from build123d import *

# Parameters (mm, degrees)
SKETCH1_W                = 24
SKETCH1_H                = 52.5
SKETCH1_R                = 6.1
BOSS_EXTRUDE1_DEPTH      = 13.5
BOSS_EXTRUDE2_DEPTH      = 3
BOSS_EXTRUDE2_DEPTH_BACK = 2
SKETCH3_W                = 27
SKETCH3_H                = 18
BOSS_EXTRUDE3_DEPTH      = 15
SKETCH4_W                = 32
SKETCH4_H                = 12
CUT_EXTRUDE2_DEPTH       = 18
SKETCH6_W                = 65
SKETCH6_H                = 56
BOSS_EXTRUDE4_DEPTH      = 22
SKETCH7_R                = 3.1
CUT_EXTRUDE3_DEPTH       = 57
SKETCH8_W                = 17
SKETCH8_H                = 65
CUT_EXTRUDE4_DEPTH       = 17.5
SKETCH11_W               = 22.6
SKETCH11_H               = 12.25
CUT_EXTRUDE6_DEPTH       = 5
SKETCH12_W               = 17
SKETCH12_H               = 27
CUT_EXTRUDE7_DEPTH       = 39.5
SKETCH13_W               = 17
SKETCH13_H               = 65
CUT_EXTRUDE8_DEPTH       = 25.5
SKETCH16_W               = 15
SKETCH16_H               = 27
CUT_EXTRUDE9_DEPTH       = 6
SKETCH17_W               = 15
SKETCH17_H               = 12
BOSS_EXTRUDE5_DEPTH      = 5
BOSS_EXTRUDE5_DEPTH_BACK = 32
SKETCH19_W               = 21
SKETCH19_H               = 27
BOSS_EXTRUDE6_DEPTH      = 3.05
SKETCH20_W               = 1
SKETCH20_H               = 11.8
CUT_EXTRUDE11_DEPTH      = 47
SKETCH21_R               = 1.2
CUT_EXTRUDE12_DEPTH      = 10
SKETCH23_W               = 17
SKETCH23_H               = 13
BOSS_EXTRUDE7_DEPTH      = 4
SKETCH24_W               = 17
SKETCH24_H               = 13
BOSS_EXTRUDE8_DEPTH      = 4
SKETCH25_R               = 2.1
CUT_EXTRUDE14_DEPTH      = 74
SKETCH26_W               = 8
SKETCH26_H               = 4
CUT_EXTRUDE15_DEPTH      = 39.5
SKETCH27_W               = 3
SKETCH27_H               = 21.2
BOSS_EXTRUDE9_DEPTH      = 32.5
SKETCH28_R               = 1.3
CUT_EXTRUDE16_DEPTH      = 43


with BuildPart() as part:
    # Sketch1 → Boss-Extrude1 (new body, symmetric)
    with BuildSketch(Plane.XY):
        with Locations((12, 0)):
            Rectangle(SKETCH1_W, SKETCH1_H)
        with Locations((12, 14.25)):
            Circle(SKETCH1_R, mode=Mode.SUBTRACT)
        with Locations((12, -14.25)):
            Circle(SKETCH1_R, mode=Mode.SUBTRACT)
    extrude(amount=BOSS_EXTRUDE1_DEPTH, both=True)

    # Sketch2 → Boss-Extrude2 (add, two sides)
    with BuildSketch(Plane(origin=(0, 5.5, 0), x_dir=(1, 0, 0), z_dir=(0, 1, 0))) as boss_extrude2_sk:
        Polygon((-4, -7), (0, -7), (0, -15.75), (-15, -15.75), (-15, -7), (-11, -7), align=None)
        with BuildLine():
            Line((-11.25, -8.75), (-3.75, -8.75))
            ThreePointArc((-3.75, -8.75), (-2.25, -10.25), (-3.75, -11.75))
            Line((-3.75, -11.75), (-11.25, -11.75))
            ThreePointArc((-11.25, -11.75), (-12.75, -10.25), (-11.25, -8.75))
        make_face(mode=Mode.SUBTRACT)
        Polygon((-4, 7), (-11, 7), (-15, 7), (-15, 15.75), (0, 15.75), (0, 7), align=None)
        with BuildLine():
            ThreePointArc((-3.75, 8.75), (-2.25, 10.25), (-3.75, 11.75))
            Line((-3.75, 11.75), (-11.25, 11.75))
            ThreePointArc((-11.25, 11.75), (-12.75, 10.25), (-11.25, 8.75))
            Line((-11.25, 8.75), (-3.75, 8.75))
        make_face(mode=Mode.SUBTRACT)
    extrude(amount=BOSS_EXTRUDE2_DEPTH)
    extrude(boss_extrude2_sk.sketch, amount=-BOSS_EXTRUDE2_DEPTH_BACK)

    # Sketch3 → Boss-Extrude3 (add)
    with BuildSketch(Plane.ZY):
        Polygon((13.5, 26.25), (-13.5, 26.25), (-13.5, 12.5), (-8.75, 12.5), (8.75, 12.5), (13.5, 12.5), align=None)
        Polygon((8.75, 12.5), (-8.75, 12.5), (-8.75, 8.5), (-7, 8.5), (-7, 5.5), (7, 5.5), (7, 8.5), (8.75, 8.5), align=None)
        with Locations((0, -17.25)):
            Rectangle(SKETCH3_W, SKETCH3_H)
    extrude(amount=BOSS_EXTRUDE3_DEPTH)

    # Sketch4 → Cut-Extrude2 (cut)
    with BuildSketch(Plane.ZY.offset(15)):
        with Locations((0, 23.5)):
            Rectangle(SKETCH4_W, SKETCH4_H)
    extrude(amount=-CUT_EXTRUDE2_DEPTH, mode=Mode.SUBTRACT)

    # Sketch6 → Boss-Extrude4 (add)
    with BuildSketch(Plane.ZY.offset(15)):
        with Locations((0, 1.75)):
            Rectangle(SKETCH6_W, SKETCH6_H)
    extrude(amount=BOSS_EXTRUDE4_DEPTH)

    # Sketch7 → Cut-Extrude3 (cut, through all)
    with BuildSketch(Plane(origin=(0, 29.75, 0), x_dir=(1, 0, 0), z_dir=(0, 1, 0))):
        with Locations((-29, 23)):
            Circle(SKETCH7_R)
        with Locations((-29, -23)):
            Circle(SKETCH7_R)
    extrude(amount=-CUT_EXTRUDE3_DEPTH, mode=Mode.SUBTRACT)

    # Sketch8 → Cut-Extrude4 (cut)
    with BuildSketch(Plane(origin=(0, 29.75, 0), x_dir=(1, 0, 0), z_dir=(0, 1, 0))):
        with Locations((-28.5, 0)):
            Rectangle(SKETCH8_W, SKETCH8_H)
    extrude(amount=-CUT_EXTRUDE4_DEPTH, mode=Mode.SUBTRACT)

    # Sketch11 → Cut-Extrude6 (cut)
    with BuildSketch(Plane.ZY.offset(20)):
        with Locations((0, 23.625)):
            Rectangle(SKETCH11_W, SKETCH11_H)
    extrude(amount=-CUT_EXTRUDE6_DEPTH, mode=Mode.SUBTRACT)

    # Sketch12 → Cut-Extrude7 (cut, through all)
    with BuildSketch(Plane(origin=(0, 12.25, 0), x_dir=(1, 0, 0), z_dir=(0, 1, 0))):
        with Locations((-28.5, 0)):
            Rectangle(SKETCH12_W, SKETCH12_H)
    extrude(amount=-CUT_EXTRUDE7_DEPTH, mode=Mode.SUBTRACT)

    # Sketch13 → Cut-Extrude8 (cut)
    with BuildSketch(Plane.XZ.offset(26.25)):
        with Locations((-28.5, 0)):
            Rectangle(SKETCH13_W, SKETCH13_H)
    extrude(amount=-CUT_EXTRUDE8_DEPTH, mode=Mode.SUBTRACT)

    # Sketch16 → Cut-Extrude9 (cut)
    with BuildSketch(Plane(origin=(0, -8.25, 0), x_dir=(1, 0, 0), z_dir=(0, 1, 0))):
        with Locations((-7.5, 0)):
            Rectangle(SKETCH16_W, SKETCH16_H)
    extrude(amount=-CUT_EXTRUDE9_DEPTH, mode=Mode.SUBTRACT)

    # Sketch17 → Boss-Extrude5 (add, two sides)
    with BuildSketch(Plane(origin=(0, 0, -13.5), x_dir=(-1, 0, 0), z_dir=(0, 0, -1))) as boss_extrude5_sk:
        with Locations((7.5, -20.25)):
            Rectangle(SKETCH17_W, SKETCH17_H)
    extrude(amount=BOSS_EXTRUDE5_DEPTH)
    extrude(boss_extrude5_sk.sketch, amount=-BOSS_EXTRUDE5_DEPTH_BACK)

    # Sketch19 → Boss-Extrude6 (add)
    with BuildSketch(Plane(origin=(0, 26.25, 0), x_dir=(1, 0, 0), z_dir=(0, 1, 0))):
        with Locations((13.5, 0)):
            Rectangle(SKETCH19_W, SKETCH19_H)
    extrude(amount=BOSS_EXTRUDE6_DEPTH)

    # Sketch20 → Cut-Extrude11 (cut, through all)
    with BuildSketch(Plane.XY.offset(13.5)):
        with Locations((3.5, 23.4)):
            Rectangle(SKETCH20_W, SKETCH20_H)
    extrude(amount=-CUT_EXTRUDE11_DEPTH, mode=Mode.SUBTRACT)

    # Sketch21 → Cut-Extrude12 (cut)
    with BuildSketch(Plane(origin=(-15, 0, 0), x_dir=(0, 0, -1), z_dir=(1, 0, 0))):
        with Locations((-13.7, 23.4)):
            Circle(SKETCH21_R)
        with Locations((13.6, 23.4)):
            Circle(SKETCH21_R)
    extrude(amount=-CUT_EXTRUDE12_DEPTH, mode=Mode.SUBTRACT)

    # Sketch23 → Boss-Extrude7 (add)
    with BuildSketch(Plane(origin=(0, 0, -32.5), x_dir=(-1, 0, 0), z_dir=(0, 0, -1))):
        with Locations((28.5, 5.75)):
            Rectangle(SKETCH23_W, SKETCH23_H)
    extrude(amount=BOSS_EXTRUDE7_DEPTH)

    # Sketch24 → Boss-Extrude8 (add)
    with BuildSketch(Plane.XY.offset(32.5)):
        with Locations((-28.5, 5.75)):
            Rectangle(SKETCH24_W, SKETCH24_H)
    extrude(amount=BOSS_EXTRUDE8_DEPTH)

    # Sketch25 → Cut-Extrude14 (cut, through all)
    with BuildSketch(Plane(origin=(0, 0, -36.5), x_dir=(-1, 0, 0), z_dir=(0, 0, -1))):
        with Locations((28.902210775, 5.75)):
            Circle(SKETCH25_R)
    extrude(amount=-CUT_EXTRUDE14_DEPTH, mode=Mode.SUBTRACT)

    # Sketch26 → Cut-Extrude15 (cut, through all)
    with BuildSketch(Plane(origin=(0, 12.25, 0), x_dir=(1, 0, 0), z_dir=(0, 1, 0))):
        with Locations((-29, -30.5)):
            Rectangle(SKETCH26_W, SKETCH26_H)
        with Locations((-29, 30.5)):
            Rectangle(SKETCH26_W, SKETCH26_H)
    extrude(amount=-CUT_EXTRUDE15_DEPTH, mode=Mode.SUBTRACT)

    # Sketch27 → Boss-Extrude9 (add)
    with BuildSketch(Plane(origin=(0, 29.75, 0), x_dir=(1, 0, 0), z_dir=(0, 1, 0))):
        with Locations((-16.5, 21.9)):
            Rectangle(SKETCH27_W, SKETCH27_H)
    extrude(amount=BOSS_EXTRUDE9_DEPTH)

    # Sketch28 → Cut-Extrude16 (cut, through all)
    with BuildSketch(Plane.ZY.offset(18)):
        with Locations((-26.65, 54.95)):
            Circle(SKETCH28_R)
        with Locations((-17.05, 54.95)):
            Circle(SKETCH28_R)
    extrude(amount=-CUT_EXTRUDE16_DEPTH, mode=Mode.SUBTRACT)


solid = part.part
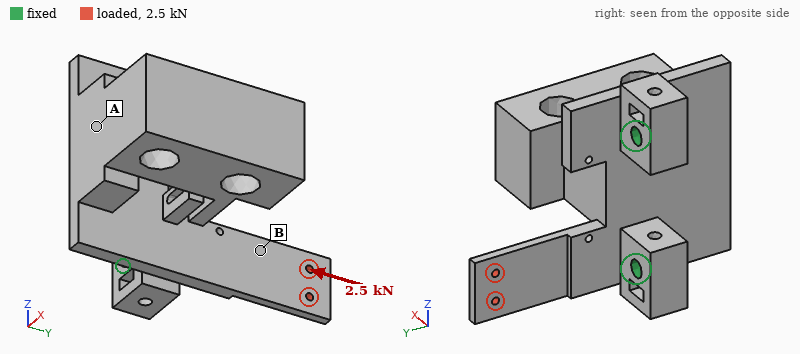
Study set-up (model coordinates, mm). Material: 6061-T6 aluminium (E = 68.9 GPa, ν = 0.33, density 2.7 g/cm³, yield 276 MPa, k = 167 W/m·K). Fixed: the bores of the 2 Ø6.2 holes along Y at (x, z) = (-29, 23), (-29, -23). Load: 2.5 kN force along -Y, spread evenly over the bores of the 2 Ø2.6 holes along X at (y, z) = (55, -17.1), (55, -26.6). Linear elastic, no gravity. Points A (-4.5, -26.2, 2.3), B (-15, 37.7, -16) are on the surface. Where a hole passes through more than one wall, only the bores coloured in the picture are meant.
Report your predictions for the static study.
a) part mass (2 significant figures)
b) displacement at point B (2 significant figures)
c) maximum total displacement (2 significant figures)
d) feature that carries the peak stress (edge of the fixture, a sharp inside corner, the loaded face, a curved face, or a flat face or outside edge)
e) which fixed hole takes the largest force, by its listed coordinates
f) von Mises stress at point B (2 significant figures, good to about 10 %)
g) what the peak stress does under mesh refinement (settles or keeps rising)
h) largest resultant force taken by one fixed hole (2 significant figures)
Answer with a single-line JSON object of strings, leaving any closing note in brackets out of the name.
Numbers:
{"part mass": "180 g", "displacement at point B": "0.078 mm", "maximum total displacement": "0.18 mm", "feature that carries the peak stress": "a sharp inside corner", "which fixed hole takes the largest force, by its listed coordinates": "(-29, -23)", "von Mises stress at point B": "40 MPa", "what the peak stress does under mesh refinement": "keeps rising", "largest resultant force taken by one fixed hole": "2.3 kN"}
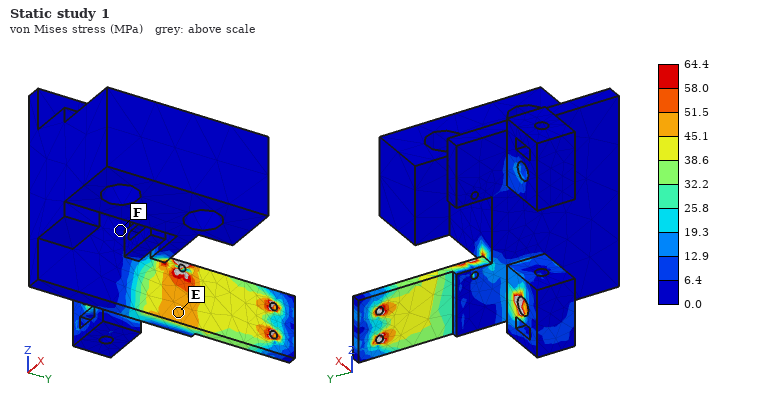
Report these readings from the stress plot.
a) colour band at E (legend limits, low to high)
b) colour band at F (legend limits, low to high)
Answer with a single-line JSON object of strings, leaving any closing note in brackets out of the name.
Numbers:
{"colour band at E": "45.1 to 51.5 MPa", "colour band at F": "0.0 to 6.4 MPa"}
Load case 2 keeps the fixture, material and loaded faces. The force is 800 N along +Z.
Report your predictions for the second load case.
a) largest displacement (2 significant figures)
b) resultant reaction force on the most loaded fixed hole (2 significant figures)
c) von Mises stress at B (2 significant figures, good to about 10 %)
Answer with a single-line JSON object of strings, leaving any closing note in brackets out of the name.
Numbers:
{"largest displacement": "0.19 mm", "resultant reaction force on the most loaded fixed hole": "800 N", "von Mises stress at B": "36 MPa"}
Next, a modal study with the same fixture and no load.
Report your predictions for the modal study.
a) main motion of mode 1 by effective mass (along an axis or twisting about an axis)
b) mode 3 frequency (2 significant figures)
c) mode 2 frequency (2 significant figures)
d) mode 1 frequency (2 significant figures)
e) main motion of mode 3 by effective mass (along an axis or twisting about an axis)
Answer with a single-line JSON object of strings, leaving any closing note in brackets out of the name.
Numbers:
{"main motion of mode 1 by effective mass": "along Y", "mode 3 frequency": "4100 Hz", "mode 2 frequency": "1700 Hz", "mode 1 frequency": "1500 Hz", "main motion of mode 3 by effective mass": "along Z"}
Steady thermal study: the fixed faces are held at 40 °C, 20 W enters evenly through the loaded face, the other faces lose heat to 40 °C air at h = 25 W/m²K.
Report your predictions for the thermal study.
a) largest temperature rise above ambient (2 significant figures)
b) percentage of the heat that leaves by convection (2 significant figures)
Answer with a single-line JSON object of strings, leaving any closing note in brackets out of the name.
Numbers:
{"largest temperature rise above ambient": "71 K", "percentage of the heat that leaves by convection": "17 %"}
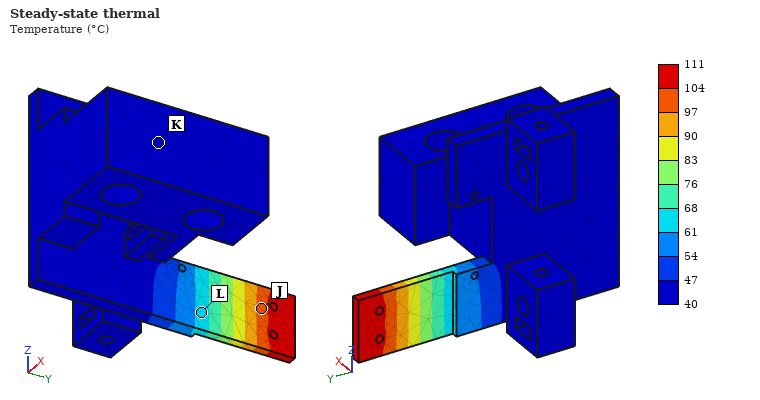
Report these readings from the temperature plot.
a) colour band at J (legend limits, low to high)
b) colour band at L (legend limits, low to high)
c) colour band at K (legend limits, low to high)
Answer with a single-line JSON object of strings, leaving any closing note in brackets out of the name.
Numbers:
{"colour band at J": "97 to 104 °C", "colour band at L": "61 to 68 °C", "colour band at K": "40 to 47 °C"}
